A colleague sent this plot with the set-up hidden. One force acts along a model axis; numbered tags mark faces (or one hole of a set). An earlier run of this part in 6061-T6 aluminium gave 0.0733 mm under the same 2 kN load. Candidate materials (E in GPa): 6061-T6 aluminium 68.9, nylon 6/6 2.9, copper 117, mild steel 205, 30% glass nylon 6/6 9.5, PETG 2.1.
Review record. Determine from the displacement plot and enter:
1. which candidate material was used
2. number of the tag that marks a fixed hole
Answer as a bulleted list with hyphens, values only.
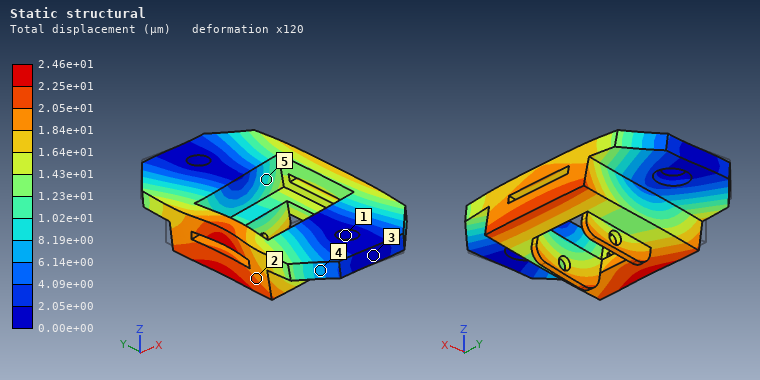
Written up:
- mild steel
- 1
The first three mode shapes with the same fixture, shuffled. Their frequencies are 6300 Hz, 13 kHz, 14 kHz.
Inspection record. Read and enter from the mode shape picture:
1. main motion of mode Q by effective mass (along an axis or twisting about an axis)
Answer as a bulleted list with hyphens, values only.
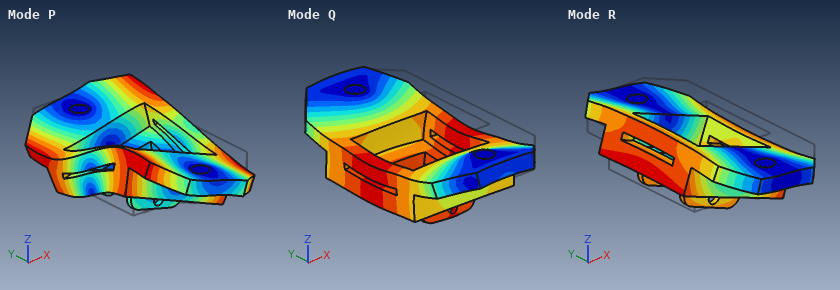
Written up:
- along Z
